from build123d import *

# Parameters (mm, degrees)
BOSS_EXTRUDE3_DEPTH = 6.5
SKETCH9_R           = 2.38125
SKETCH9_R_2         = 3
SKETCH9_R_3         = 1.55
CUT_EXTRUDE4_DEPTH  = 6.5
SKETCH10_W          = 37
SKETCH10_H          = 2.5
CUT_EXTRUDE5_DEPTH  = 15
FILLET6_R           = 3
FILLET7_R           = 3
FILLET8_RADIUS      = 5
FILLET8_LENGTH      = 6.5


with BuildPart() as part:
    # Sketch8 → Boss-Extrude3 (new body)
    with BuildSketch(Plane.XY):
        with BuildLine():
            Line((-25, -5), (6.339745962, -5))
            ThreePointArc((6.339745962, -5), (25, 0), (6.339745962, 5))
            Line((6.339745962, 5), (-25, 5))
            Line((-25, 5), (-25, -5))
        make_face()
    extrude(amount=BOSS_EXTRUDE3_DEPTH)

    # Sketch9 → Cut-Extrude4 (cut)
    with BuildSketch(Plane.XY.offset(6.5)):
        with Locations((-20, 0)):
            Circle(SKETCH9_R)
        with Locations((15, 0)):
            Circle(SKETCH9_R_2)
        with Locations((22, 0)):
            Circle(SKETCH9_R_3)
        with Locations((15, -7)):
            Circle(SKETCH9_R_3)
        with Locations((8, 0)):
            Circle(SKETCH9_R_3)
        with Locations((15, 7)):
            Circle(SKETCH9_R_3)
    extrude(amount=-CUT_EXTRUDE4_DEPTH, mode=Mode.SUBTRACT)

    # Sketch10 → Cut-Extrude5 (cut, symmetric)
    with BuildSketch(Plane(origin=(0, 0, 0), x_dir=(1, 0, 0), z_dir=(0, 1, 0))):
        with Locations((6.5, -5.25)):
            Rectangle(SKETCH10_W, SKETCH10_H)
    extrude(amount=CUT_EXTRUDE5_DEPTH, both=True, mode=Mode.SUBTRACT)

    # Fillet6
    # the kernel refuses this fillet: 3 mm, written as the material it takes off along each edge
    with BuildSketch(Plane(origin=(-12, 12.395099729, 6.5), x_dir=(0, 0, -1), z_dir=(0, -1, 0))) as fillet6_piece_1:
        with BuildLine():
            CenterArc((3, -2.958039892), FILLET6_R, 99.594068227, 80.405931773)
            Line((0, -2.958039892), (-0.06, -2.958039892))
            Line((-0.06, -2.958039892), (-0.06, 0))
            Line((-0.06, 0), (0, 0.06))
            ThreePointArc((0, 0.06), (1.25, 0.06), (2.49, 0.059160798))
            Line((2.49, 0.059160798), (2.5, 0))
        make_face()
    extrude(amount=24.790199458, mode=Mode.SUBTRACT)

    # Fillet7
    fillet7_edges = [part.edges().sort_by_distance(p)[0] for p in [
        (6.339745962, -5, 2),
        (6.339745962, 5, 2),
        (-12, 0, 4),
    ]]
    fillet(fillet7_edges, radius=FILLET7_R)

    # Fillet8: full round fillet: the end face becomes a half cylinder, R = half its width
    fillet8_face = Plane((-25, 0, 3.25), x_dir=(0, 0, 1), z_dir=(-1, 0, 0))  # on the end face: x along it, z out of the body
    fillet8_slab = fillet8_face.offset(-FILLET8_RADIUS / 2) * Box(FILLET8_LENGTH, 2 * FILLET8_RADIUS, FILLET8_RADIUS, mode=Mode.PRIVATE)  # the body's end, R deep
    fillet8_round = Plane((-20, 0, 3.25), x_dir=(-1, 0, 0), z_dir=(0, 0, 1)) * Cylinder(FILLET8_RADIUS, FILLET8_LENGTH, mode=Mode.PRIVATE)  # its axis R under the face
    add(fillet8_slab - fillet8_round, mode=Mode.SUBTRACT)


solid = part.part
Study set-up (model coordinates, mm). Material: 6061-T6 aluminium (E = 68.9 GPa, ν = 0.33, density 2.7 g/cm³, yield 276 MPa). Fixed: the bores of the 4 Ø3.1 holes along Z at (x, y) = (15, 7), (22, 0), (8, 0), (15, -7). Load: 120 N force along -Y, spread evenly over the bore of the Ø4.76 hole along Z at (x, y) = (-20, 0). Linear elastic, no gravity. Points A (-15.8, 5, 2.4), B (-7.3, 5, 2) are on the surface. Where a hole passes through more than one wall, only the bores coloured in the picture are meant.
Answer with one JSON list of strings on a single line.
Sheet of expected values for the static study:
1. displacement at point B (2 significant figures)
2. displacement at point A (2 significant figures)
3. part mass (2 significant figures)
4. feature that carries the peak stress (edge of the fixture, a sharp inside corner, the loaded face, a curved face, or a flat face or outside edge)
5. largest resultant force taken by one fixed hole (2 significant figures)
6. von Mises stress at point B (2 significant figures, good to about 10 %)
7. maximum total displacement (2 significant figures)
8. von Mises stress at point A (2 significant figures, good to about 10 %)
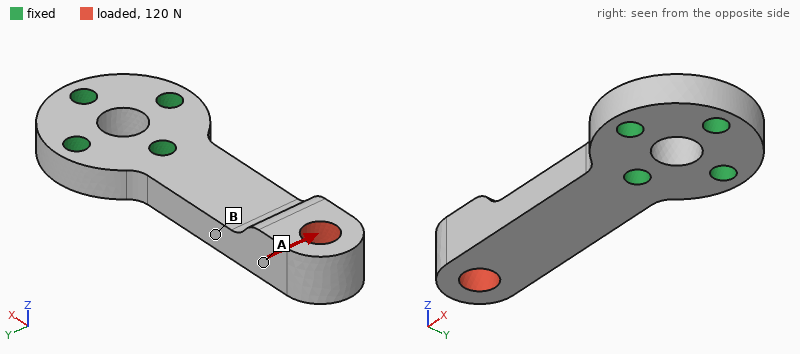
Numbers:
["20 µm", "37 µm", "6.4 g", "a curved face", "200 N", "23 MPa", "58 µm", "7.5 MPa"]
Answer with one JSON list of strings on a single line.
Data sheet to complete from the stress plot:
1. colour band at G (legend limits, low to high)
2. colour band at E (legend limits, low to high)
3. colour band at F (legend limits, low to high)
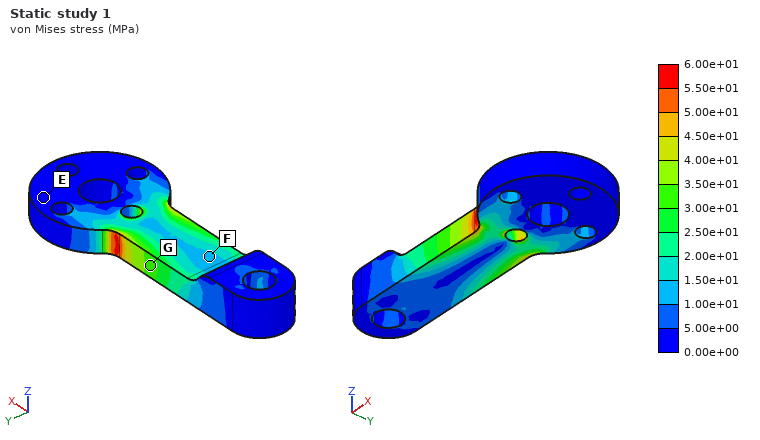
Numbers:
["3.00e+01 to 3.50e+01 MPa", "0.00e+00 to 5.00e+00 MPa", "1.00e+01 to 1.50e+01 MPa"]
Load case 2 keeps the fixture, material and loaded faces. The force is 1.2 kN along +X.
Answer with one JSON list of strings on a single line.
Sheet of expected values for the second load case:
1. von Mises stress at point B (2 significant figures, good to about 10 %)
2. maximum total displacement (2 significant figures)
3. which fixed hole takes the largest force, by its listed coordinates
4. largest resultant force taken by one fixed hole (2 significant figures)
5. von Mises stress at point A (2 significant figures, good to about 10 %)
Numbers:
["29 MPa", "0.19 mm", "(8, 0)", "920 N", "28 MPa"]
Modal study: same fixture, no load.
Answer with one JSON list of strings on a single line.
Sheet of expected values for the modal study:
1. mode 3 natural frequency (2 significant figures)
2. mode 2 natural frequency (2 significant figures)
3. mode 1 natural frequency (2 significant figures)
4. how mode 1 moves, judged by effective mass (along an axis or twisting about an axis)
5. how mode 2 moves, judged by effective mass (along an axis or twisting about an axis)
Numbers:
["14 kHz", "6300 Hz", "2900 Hz", "along Z", "along Y"]
